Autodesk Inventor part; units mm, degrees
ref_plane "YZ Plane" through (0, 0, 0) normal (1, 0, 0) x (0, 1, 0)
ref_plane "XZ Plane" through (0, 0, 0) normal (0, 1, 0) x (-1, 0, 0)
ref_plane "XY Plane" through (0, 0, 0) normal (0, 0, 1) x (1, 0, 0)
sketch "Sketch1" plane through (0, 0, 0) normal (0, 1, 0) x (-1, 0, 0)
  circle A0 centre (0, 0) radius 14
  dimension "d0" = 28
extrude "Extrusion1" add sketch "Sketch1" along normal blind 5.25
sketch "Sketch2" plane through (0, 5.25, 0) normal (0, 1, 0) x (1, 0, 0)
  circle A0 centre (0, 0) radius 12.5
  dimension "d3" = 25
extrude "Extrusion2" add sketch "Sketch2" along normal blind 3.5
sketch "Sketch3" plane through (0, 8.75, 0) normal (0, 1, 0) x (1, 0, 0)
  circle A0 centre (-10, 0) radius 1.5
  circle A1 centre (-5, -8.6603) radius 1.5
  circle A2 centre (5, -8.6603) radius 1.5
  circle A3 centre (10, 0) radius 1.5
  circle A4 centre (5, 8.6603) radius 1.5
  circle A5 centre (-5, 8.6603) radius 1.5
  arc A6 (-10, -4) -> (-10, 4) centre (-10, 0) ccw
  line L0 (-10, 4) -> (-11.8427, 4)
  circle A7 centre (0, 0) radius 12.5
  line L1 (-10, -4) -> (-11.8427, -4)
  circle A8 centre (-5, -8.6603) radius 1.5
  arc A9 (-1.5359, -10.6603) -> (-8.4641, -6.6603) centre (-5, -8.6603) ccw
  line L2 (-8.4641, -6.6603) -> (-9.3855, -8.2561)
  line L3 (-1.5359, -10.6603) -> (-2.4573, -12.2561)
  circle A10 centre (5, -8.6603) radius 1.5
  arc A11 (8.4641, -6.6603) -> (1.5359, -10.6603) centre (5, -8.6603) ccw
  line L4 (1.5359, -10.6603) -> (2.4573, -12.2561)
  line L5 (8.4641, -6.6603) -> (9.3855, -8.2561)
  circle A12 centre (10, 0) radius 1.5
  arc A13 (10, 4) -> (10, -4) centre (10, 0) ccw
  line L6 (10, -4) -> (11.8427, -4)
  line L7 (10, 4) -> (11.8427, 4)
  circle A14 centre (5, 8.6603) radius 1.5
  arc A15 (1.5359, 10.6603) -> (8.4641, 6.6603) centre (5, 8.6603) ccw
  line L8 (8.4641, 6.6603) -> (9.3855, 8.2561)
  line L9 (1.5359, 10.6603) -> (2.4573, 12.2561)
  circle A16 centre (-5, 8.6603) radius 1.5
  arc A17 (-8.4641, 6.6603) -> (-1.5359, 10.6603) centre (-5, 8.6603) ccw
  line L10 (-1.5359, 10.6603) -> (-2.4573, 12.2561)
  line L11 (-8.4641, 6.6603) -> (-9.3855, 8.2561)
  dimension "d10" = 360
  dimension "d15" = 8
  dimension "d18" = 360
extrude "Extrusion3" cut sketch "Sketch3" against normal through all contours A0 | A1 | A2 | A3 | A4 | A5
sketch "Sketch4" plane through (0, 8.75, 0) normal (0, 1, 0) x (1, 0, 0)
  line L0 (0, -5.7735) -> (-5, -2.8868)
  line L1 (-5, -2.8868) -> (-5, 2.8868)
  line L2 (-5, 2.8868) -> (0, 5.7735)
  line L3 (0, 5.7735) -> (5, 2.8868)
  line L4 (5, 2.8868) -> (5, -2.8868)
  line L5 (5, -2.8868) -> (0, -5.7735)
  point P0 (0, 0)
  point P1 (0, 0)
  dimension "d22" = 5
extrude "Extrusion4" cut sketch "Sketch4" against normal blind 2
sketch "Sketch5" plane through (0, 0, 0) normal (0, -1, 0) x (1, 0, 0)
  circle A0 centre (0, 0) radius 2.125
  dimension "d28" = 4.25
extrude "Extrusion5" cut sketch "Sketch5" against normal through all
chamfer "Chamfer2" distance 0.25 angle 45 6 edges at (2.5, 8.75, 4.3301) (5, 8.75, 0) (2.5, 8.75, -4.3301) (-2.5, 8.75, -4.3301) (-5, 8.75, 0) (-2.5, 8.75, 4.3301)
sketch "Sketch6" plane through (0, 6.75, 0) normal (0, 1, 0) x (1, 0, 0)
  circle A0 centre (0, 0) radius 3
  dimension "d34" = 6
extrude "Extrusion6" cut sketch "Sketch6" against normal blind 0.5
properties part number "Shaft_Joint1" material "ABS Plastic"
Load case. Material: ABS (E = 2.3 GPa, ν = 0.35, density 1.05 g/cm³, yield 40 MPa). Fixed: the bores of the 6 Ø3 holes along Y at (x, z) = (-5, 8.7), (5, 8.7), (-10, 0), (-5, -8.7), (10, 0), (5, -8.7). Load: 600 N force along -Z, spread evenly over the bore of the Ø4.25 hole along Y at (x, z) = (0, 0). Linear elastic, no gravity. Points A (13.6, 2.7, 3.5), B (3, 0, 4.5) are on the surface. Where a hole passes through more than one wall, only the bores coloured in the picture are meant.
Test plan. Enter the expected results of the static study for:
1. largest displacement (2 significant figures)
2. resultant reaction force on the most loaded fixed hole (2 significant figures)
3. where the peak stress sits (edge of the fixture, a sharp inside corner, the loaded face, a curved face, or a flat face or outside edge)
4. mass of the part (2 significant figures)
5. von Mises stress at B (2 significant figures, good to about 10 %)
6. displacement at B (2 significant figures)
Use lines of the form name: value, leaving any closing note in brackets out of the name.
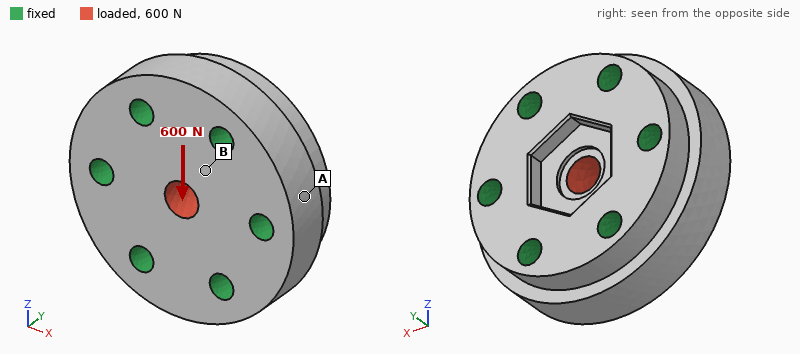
largest displacement: 17 µm
resultant reaction force on the most loaded fixed hole: 150 N
where the peak stress sits: a sharp inside corner
mass of the part: 4.5 g
von Mises stress at B: 4.6 MPa
displacement at B: 6.9 µm
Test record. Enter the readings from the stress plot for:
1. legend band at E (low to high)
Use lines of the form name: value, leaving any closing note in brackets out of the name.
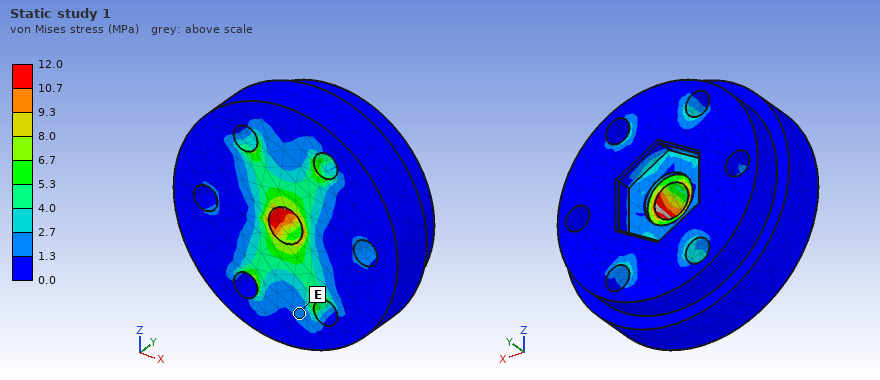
legend band at E: 1.3 to 2.7 MPa
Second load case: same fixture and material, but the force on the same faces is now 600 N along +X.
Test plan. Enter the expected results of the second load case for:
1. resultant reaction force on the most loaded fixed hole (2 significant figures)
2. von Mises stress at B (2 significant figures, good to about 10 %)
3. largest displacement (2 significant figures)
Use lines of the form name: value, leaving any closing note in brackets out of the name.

resultant reaction force on the most loaded fixed hole: 170 N
von Mises stress at B: 2.9 MPa
largest displacement: 17 µm
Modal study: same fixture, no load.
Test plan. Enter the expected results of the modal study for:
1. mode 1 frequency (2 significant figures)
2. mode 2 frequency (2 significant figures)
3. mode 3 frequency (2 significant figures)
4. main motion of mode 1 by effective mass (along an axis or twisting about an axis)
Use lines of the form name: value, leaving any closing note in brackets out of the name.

mode 1 frequency: 32 kHz
mode 2 frequency: 39 kHz
mode 3 frequency: 39 kHz
main motion of mode 1 by effective mass: along Y
